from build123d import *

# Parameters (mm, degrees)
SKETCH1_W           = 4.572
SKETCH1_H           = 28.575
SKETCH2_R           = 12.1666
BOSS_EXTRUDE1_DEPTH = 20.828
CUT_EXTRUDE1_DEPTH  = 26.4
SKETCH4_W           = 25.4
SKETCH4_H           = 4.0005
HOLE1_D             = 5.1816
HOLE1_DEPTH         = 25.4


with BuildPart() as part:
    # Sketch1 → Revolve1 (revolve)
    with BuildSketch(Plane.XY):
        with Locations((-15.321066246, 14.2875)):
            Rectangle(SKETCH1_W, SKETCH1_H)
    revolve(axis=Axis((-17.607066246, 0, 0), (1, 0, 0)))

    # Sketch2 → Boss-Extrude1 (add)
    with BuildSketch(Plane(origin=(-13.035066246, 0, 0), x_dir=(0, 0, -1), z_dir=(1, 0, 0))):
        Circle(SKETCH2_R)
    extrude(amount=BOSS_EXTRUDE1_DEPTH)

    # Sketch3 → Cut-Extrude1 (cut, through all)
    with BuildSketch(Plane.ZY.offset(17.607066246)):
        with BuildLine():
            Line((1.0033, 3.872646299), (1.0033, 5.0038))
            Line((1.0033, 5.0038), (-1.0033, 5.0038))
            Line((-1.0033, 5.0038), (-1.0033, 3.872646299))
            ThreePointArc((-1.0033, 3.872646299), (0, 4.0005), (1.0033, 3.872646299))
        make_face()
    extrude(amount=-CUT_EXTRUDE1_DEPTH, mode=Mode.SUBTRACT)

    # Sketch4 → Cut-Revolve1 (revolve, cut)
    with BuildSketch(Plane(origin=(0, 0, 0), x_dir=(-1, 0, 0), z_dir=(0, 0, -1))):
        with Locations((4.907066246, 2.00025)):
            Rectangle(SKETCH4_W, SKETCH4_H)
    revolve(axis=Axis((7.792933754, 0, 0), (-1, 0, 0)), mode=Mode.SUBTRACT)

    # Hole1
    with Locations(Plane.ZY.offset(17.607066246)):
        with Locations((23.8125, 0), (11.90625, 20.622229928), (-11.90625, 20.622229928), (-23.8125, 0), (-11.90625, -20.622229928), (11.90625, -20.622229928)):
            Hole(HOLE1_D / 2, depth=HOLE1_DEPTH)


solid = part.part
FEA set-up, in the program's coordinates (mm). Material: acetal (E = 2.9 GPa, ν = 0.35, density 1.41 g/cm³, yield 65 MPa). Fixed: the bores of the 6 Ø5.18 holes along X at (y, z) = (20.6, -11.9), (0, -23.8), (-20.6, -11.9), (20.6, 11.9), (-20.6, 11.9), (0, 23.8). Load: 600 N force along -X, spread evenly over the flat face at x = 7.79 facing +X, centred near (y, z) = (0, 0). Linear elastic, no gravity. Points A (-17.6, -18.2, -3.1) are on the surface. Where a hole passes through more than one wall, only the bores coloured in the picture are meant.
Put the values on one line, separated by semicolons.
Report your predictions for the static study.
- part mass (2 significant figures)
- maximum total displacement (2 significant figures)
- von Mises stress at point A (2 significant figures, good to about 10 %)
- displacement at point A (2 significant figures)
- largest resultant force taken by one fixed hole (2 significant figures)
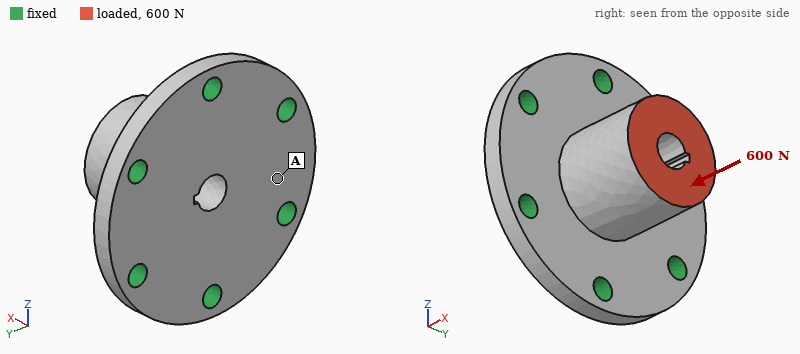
28 g; 77 µm; 3.1 MPa; 27 µm; 110 N
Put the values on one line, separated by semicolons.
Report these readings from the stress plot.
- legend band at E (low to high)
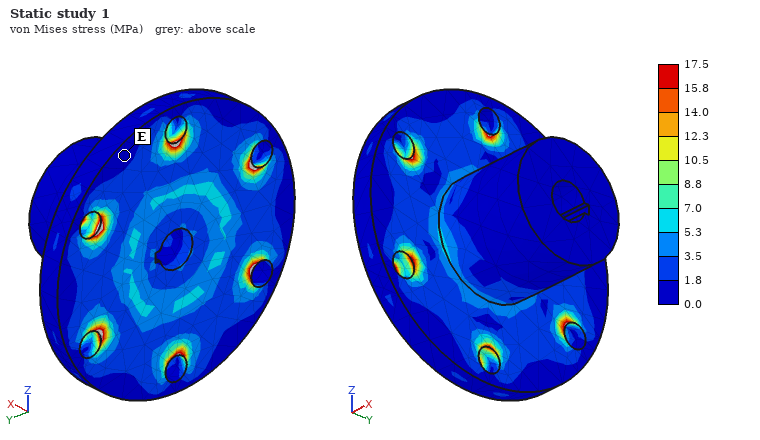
0.0 to 1.8 MPa
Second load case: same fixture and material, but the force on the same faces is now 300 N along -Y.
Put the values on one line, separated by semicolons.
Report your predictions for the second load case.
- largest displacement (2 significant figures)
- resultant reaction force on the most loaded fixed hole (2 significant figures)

0.16 mm; 130 N
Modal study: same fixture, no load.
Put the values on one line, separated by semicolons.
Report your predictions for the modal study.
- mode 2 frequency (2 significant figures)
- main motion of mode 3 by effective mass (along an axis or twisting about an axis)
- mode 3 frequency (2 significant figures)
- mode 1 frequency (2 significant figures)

3200 Hz; along X; 3600 Hz; 3100 Hz
